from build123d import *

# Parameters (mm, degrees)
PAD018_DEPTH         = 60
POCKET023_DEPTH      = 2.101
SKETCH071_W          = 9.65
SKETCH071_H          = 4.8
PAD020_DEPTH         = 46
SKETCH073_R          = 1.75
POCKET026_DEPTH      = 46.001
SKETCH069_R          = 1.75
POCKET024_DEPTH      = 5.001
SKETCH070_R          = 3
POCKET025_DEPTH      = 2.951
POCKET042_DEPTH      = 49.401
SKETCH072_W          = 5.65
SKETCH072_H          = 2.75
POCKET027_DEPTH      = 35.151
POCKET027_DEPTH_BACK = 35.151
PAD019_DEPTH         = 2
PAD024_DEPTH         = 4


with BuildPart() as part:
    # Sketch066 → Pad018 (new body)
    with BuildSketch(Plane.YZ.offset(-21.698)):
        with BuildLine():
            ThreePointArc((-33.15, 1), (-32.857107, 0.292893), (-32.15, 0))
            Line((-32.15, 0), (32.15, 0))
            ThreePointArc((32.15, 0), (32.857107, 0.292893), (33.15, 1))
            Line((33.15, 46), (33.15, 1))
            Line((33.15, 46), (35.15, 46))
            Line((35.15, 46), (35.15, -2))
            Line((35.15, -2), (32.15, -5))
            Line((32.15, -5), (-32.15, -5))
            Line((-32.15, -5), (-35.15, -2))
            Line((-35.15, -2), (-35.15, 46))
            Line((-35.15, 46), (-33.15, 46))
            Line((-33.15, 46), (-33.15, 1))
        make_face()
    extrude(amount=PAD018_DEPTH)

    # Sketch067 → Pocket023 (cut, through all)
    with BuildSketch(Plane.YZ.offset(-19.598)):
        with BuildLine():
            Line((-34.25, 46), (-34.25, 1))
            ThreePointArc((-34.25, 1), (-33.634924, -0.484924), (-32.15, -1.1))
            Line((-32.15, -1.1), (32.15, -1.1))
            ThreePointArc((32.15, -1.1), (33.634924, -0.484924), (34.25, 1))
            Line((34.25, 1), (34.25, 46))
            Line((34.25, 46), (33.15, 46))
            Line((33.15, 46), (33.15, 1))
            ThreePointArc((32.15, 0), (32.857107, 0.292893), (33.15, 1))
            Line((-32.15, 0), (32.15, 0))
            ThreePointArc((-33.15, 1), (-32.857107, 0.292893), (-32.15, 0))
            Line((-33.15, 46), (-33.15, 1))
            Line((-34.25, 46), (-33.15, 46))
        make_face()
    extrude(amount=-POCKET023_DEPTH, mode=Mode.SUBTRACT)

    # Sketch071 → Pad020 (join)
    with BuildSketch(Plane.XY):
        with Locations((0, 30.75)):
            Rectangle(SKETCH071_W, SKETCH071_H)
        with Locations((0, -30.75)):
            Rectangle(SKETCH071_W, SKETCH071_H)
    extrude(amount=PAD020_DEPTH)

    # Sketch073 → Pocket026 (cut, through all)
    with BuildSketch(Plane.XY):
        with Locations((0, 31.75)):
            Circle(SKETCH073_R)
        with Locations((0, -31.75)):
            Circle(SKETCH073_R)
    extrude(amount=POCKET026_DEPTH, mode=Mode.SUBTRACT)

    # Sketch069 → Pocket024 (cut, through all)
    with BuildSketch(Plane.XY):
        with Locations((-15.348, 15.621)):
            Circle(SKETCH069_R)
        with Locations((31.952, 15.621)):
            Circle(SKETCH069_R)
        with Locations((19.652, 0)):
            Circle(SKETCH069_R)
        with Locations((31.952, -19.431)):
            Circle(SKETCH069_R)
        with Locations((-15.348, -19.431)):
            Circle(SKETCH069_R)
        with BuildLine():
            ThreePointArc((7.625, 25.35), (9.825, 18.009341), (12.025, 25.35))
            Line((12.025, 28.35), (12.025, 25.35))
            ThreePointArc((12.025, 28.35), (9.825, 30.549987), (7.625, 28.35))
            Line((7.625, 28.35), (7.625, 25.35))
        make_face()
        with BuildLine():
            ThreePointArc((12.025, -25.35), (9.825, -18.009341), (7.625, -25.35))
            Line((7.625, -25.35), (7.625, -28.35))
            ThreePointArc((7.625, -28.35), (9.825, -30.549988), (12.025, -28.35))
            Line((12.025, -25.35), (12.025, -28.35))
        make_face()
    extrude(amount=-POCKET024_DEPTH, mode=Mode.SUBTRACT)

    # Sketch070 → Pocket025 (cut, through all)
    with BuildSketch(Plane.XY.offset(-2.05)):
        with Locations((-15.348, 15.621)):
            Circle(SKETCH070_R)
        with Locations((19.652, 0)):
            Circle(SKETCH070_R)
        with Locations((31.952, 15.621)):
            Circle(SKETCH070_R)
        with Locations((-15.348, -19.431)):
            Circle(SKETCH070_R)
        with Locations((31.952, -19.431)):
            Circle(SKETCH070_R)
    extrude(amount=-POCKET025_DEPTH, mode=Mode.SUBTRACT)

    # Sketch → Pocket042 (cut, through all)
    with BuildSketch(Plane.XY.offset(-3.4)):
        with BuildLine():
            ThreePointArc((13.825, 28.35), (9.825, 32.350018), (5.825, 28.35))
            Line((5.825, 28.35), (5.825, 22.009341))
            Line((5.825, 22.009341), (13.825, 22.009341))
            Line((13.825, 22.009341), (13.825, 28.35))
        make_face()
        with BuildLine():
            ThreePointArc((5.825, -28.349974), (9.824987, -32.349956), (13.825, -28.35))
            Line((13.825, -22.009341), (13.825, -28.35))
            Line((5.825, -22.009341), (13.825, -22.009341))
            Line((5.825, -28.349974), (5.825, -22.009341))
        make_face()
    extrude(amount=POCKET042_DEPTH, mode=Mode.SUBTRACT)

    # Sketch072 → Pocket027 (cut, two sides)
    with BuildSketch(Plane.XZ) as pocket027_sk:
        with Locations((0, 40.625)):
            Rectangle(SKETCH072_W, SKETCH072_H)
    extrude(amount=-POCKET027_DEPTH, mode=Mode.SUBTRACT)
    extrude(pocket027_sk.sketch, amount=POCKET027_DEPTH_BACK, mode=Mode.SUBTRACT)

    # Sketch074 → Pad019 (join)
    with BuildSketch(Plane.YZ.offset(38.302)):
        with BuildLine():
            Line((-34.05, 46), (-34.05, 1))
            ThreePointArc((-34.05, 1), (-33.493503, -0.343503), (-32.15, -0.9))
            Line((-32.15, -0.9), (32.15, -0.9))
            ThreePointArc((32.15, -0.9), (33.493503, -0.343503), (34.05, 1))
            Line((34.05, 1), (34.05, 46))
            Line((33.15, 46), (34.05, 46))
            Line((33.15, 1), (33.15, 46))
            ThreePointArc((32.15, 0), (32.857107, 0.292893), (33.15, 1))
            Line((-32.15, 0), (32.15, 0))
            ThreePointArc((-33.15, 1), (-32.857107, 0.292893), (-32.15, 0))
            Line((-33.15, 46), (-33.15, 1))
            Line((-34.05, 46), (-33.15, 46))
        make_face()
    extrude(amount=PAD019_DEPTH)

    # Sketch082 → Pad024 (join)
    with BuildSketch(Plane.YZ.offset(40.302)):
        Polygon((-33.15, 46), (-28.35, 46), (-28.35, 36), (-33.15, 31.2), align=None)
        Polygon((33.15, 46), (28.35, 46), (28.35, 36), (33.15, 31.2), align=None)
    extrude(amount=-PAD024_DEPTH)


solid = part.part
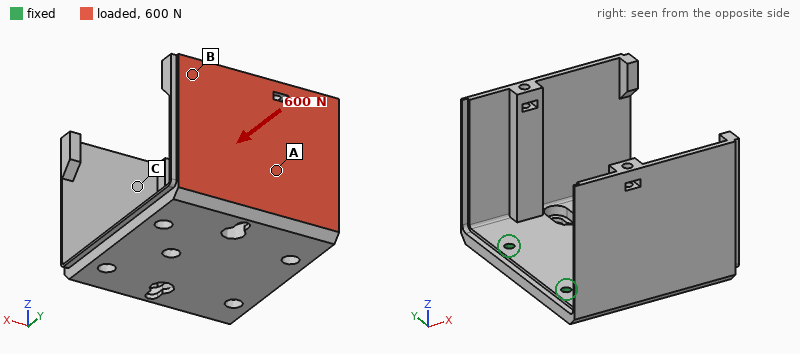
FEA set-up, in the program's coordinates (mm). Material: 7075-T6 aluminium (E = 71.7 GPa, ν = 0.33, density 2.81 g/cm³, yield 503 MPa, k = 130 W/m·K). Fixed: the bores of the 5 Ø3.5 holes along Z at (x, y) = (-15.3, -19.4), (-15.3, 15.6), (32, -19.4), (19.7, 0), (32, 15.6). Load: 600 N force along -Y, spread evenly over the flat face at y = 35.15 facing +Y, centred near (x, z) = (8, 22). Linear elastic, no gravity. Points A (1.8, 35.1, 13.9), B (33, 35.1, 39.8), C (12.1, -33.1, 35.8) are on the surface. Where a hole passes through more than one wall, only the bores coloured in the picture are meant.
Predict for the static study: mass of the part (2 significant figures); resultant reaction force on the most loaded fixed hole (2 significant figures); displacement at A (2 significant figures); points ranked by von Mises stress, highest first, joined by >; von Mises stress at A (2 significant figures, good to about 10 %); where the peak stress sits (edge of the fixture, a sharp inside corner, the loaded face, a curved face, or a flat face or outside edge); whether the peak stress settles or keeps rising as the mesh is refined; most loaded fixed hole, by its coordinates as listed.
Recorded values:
95 g
760 N
0.22 mm
A > B > C
37 MPa
edge of the fixture
keeps rising
(-15.3, 15.6)
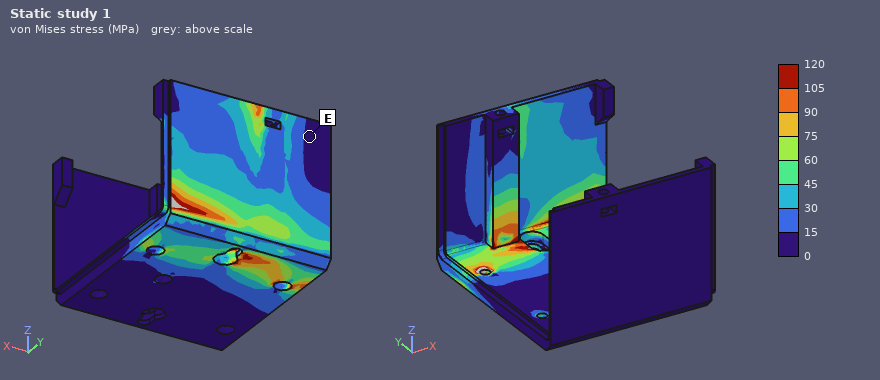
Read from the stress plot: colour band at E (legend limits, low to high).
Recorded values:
0 to 15 MPa
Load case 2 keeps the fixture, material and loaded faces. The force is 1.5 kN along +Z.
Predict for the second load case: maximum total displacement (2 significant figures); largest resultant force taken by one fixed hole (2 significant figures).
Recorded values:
0.66 mm
1.6 kN
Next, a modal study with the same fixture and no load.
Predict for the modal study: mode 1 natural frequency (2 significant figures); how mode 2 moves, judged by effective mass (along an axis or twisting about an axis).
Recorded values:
1100 Hz
along Y
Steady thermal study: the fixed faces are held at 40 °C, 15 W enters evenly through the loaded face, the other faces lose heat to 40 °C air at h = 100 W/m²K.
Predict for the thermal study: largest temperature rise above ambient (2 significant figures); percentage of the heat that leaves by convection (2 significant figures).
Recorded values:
16 K
49 %
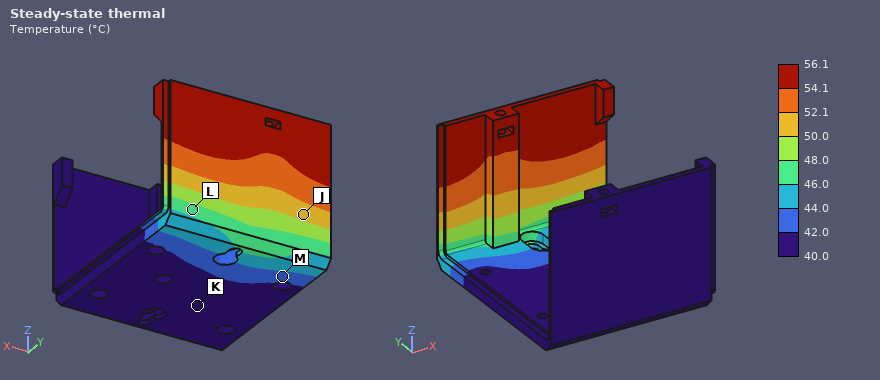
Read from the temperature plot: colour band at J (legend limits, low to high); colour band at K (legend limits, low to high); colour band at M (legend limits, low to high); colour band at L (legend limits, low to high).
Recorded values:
50.0 to 52.1 °C
40.0 to 42.0 °C
42.0 to 44.0 °C
46.0 to 48.0 °C
